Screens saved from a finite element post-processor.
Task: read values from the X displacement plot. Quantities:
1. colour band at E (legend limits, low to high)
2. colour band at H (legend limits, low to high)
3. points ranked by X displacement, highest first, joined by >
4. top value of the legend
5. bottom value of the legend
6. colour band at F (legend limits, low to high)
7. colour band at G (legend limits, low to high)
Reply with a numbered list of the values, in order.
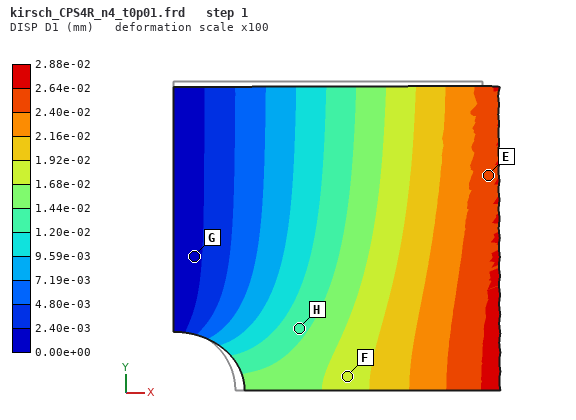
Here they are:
1. 2.40e-02 to 2.64e-02 mm
2. 1.20e-02 to 1.44e-02 mm
3. E > F > H > G
4. 2.88e-02 mm
5. 0.00e+00 mm
6. 1.68e-02 to 1.92e-02 mm
7. 0.00e+00 to 2.40e-03 mm
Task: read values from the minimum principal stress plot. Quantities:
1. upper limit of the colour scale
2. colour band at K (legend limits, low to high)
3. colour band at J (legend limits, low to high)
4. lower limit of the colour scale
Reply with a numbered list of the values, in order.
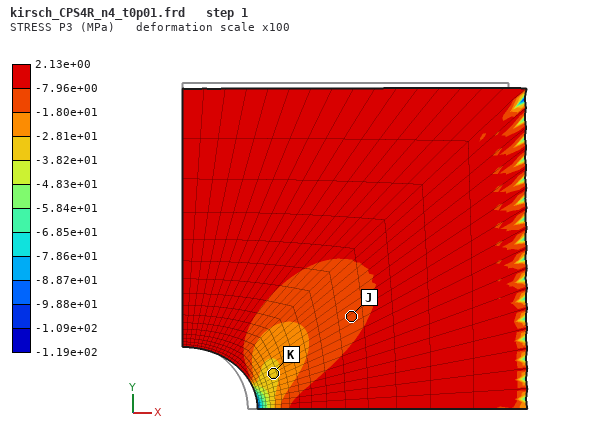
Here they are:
1. 2.13e+00 MPa
2. -3.82e+01 to -2.81e+01 MPa
3. -1.80e+01 to -7.96e+00 MPa
4. -1.19e+02 MPa
